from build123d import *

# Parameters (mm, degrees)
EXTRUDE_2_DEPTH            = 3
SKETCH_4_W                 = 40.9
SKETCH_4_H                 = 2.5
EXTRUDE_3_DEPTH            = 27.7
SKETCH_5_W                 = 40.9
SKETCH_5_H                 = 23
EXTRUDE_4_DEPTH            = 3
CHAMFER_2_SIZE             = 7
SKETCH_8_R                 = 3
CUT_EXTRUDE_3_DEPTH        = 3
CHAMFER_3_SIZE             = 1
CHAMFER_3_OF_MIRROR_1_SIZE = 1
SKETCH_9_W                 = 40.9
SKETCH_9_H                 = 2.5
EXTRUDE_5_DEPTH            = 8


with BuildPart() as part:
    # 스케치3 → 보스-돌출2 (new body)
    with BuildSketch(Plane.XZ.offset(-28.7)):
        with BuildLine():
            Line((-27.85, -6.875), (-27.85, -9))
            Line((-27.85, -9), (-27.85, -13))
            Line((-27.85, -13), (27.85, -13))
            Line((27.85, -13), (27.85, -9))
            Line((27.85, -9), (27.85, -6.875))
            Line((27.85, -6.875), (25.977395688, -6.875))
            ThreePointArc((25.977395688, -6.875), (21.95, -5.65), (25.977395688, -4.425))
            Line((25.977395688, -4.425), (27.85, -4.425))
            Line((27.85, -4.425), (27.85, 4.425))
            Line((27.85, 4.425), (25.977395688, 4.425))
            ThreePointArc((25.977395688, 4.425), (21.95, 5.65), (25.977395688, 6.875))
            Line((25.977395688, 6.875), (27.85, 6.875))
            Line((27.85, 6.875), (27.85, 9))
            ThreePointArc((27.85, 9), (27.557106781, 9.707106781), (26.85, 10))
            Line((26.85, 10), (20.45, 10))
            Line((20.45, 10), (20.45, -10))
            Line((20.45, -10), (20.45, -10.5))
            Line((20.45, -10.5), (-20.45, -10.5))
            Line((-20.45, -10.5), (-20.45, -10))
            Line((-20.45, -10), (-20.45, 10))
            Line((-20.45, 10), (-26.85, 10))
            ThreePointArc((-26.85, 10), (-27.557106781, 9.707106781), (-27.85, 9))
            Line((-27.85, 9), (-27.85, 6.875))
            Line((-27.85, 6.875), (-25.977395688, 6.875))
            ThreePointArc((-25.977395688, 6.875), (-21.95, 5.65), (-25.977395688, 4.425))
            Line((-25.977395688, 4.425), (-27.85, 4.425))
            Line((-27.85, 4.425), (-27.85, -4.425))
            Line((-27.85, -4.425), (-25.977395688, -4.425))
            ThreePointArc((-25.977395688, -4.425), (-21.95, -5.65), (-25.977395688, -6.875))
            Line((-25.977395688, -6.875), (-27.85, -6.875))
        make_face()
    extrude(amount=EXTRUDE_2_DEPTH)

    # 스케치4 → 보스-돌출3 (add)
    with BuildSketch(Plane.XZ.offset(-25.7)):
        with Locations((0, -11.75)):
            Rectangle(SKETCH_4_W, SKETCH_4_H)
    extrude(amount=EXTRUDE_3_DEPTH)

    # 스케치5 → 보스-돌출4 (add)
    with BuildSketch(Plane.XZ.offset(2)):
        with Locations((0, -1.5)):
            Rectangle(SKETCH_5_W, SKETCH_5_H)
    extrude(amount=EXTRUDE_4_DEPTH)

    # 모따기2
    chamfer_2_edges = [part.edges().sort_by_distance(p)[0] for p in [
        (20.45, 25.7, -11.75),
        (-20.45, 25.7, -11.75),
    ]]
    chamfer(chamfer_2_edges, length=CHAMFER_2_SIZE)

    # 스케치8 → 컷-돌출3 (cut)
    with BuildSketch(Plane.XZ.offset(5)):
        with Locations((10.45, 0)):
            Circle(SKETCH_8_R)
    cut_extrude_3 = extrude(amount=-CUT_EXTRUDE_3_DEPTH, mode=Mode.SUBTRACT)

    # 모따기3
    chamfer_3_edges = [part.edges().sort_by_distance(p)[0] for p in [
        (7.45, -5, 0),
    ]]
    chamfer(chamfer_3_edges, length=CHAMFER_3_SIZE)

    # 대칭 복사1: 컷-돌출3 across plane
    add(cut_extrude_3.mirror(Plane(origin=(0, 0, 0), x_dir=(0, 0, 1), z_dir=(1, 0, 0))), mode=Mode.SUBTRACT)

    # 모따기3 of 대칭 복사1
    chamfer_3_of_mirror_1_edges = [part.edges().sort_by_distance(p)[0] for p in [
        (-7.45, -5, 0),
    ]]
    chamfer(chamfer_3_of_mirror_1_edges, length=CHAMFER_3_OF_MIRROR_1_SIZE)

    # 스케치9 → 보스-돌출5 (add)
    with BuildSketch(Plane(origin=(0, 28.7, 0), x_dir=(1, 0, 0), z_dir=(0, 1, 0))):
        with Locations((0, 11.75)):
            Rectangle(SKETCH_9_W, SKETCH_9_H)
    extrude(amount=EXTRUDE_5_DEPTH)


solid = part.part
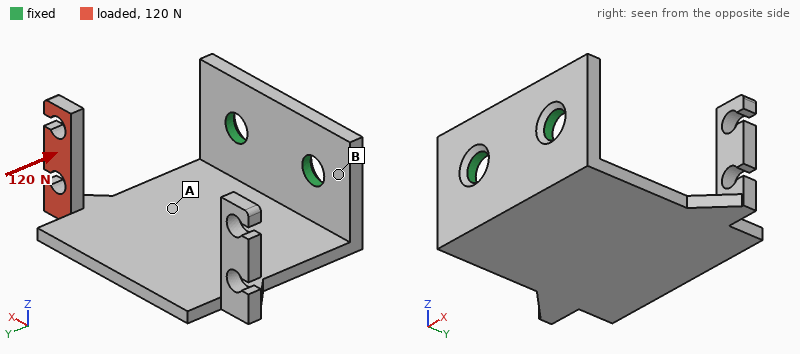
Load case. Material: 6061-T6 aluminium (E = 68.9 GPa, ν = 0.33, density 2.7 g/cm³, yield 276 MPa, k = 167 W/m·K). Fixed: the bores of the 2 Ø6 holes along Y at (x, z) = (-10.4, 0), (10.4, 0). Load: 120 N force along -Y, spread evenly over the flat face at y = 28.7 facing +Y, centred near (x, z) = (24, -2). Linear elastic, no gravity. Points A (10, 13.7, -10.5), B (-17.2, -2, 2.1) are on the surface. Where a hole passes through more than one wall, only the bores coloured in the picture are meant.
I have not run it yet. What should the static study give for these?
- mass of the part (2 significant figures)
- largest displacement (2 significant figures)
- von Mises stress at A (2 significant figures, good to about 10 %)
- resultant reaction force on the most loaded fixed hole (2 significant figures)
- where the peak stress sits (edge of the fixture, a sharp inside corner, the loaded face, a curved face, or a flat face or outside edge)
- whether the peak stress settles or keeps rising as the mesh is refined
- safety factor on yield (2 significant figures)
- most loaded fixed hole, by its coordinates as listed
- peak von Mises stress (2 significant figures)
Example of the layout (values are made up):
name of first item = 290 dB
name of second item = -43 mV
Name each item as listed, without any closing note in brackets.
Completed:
mass of the part = 20 g
largest displacement = 0.86 mm
von Mises stress at A = 36 MPa
resultant reaction force on the most loaded fixed hole = 170 N
where the peak stress sits = a curved face
whether the peak stress settles or keeps rising as the mesh is refined = settles
safety factor on yield = 0.74
most loaded fixed hole, by its coordinates as listed = (10.4, 0)
peak von Mises stress = 370 MPa
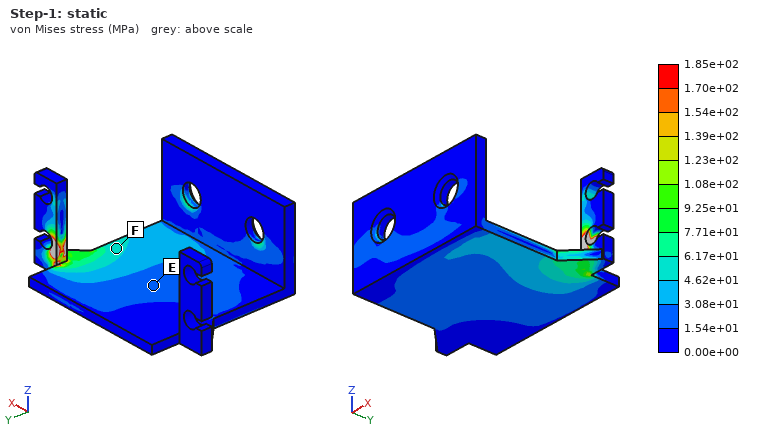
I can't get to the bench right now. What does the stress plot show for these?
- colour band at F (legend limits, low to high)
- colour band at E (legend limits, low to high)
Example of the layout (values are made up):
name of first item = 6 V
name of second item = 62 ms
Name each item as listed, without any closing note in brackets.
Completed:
colour band at F = 4.62e+01 to 6.17e+01 MPa
colour band at E = 1.54e+01 to 3.08e+01 MPa
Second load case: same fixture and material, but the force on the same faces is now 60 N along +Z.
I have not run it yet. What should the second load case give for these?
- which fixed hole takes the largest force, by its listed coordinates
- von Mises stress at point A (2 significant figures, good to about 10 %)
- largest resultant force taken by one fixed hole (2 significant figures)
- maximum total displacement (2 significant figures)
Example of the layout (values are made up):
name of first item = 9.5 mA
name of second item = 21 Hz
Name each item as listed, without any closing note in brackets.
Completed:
which fixed hole takes the largest force, by its listed coordinates = (10.4, 0)
von Mises stress at point A = 34 MPa
largest resultant force taken by one fixed hole = 91 N
maximum total displacement = 0.67 mm
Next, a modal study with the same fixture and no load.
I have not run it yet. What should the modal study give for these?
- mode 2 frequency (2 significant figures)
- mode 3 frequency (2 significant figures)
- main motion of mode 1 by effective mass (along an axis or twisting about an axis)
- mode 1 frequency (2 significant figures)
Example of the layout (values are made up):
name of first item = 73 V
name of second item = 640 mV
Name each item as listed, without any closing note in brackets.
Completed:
mode 2 frequency = 1400 Hz
mode 3 frequency = 2000 Hz
main motion of mode 1 by effective mass = along Z
mode 1 frequency = 860 Hz
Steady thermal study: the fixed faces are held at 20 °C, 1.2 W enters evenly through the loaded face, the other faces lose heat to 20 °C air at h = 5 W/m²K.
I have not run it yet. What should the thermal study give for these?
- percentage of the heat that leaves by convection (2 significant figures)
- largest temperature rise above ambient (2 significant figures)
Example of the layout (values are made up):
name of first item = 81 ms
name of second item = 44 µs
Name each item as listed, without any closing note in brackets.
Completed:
percentage of the heat that leaves by convection = 5.0 %
largest temperature rise above ambient = 14 K
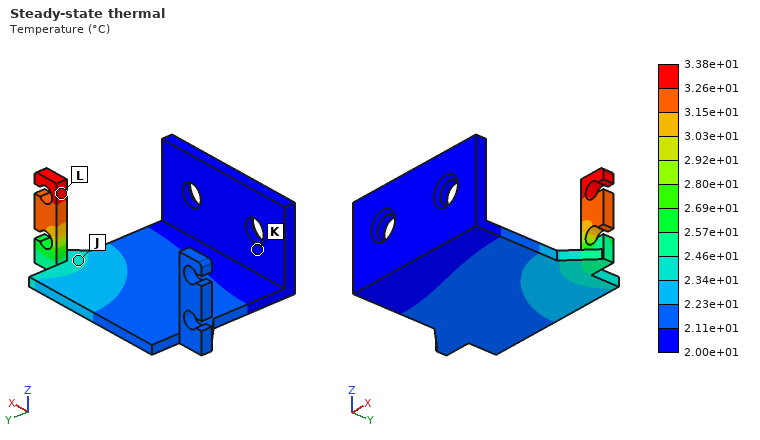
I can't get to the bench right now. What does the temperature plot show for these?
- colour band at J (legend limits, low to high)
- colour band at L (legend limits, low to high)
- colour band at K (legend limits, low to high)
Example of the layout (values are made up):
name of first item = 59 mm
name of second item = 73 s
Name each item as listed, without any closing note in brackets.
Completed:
colour band at J = 2.34e+01 to 2.46e+01 °C
colour band at L = 3.26e+01 to 3.38e+01 °C
colour band at K = 2.00e+01 to 2.11e+01 °C
